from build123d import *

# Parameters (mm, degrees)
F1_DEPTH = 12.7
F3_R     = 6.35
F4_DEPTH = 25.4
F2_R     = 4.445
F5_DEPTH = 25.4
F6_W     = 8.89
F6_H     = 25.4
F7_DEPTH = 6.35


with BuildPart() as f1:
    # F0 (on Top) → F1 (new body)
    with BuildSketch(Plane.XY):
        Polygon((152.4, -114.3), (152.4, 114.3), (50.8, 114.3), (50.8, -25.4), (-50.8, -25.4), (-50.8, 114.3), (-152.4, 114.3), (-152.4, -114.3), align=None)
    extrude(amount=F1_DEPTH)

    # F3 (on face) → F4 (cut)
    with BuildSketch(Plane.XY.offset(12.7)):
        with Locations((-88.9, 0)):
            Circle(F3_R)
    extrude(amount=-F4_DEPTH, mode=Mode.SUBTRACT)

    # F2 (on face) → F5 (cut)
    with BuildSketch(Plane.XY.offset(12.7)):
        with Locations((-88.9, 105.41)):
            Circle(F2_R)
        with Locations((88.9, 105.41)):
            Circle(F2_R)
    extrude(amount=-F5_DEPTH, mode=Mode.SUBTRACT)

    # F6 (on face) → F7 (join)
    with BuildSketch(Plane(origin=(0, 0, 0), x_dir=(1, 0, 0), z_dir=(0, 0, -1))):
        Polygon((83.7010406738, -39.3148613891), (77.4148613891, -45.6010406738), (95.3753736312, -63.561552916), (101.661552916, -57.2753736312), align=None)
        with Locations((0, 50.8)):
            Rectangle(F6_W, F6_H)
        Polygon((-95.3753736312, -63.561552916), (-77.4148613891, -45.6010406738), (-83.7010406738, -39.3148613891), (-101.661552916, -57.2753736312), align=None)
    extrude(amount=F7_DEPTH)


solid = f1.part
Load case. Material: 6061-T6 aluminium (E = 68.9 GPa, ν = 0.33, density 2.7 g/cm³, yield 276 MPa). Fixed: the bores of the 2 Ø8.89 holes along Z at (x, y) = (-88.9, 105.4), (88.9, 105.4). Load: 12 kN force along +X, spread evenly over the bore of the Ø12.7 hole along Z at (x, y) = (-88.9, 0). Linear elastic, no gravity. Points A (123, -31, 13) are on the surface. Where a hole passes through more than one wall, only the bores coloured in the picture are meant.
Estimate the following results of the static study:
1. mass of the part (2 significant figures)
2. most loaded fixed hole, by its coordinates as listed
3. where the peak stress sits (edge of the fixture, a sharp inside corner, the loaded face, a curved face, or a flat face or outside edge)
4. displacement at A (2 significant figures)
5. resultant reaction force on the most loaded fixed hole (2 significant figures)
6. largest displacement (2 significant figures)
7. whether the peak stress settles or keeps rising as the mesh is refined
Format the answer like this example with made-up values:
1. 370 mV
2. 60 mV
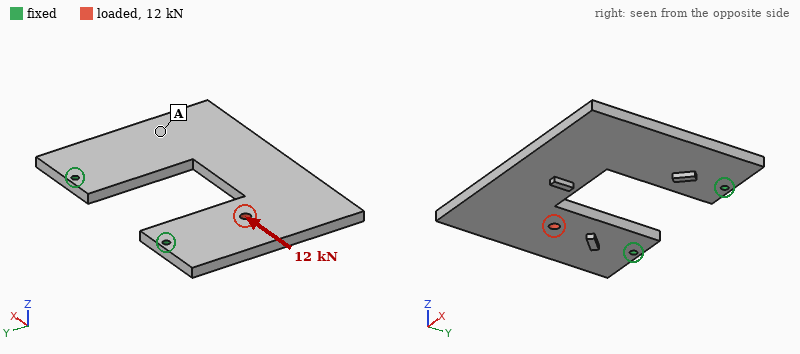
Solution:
1. 1.9 kg
2. (-88.9, 105.4)
3. edge of the fixture
4. 0.18 mm
5. 9.9 kN
6. 0.25 mm
7. keeps rising
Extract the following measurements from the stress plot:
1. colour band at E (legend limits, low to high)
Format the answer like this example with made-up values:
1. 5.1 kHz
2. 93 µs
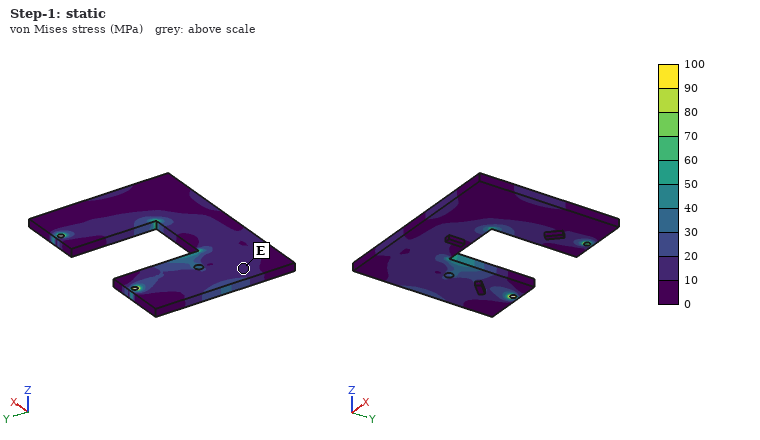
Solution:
1. 10 to 20 MPa
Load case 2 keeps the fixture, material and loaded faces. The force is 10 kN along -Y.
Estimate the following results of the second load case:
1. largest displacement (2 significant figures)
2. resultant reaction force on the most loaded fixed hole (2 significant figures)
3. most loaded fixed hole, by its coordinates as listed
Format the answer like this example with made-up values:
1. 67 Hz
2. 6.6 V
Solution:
1. 38 µm
2. 9.9 kN
3. (-88.9, 105.4)
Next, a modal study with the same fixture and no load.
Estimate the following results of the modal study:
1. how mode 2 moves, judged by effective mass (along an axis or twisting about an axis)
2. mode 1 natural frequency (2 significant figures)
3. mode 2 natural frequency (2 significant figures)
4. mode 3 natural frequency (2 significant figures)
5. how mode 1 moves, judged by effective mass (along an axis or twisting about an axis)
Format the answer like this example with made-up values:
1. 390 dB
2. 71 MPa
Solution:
1. twisting about Y
2. 150 Hz
3. 310 Hz
4. 800 Hz
5. along Z
